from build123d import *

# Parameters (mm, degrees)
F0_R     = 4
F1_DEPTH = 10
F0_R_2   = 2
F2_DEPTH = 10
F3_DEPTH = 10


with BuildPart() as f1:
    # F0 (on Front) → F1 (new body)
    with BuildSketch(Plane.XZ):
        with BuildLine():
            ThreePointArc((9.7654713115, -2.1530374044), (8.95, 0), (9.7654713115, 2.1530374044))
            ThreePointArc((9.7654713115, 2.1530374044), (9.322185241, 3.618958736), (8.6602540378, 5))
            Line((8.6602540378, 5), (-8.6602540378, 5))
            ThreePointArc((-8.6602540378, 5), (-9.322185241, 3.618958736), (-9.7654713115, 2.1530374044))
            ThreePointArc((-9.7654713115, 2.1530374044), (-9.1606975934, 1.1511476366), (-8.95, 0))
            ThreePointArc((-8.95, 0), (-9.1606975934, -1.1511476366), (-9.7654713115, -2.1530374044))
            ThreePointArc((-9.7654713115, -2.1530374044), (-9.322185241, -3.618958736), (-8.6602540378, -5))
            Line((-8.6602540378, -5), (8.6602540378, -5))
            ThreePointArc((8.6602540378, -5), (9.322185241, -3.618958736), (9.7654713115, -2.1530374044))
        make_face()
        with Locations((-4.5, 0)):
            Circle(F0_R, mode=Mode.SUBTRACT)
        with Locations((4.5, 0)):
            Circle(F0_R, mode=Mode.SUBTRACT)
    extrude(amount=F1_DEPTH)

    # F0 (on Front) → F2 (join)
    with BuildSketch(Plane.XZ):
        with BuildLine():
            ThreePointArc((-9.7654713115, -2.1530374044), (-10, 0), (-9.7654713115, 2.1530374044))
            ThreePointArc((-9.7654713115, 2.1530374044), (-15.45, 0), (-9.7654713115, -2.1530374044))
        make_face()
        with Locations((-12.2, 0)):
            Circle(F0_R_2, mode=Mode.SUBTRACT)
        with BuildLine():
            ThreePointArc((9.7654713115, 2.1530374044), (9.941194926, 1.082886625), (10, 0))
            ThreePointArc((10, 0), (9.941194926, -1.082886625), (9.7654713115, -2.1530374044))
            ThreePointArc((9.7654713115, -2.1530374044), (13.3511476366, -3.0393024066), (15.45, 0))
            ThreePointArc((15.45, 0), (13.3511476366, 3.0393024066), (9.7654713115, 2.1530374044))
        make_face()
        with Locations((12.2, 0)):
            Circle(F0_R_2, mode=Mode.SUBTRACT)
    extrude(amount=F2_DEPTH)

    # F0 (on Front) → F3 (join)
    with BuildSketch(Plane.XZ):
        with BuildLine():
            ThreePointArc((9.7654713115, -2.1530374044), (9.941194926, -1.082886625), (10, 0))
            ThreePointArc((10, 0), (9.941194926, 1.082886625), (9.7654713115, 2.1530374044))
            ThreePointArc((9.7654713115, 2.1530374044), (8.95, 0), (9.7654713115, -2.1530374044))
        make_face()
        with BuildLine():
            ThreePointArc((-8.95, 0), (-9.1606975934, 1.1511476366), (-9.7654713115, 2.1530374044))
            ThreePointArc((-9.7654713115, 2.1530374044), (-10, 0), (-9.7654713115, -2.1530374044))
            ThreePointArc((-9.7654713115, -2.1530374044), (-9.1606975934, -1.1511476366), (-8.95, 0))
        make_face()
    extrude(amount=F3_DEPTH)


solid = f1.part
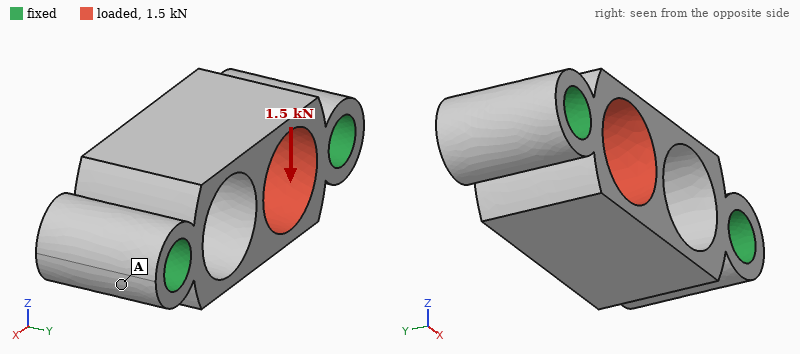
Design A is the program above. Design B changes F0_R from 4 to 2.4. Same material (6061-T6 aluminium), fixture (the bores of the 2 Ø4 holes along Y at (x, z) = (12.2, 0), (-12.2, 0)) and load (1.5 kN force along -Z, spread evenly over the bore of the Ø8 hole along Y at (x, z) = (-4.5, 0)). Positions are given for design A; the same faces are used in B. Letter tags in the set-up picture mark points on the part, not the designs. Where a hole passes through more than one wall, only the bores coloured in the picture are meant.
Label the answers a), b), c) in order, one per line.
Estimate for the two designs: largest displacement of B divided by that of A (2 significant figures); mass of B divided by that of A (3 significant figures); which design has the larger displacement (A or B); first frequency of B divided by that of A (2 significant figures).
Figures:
a) 0.24
b) 1.51
c) A
d) 1.6
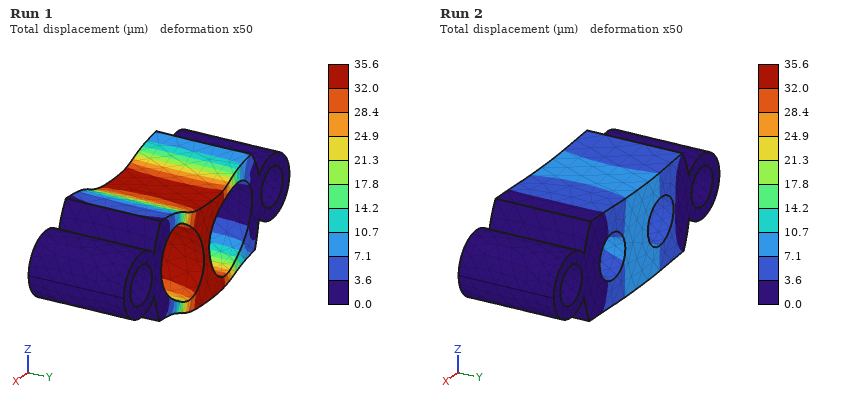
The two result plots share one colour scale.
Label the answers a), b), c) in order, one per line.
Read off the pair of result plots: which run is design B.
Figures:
a) Run 2
